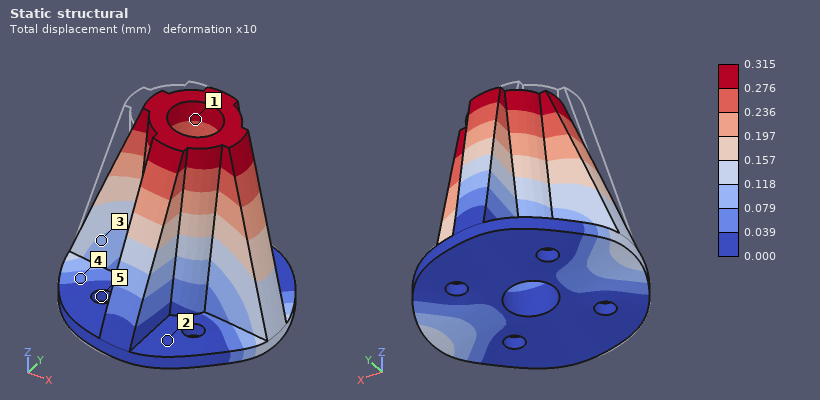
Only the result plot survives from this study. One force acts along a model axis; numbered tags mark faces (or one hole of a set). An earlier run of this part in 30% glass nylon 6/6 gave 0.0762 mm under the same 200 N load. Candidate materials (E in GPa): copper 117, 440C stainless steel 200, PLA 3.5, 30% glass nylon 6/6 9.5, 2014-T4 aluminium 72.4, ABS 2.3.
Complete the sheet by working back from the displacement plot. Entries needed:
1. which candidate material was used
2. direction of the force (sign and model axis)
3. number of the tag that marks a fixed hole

ABS
+X
5
